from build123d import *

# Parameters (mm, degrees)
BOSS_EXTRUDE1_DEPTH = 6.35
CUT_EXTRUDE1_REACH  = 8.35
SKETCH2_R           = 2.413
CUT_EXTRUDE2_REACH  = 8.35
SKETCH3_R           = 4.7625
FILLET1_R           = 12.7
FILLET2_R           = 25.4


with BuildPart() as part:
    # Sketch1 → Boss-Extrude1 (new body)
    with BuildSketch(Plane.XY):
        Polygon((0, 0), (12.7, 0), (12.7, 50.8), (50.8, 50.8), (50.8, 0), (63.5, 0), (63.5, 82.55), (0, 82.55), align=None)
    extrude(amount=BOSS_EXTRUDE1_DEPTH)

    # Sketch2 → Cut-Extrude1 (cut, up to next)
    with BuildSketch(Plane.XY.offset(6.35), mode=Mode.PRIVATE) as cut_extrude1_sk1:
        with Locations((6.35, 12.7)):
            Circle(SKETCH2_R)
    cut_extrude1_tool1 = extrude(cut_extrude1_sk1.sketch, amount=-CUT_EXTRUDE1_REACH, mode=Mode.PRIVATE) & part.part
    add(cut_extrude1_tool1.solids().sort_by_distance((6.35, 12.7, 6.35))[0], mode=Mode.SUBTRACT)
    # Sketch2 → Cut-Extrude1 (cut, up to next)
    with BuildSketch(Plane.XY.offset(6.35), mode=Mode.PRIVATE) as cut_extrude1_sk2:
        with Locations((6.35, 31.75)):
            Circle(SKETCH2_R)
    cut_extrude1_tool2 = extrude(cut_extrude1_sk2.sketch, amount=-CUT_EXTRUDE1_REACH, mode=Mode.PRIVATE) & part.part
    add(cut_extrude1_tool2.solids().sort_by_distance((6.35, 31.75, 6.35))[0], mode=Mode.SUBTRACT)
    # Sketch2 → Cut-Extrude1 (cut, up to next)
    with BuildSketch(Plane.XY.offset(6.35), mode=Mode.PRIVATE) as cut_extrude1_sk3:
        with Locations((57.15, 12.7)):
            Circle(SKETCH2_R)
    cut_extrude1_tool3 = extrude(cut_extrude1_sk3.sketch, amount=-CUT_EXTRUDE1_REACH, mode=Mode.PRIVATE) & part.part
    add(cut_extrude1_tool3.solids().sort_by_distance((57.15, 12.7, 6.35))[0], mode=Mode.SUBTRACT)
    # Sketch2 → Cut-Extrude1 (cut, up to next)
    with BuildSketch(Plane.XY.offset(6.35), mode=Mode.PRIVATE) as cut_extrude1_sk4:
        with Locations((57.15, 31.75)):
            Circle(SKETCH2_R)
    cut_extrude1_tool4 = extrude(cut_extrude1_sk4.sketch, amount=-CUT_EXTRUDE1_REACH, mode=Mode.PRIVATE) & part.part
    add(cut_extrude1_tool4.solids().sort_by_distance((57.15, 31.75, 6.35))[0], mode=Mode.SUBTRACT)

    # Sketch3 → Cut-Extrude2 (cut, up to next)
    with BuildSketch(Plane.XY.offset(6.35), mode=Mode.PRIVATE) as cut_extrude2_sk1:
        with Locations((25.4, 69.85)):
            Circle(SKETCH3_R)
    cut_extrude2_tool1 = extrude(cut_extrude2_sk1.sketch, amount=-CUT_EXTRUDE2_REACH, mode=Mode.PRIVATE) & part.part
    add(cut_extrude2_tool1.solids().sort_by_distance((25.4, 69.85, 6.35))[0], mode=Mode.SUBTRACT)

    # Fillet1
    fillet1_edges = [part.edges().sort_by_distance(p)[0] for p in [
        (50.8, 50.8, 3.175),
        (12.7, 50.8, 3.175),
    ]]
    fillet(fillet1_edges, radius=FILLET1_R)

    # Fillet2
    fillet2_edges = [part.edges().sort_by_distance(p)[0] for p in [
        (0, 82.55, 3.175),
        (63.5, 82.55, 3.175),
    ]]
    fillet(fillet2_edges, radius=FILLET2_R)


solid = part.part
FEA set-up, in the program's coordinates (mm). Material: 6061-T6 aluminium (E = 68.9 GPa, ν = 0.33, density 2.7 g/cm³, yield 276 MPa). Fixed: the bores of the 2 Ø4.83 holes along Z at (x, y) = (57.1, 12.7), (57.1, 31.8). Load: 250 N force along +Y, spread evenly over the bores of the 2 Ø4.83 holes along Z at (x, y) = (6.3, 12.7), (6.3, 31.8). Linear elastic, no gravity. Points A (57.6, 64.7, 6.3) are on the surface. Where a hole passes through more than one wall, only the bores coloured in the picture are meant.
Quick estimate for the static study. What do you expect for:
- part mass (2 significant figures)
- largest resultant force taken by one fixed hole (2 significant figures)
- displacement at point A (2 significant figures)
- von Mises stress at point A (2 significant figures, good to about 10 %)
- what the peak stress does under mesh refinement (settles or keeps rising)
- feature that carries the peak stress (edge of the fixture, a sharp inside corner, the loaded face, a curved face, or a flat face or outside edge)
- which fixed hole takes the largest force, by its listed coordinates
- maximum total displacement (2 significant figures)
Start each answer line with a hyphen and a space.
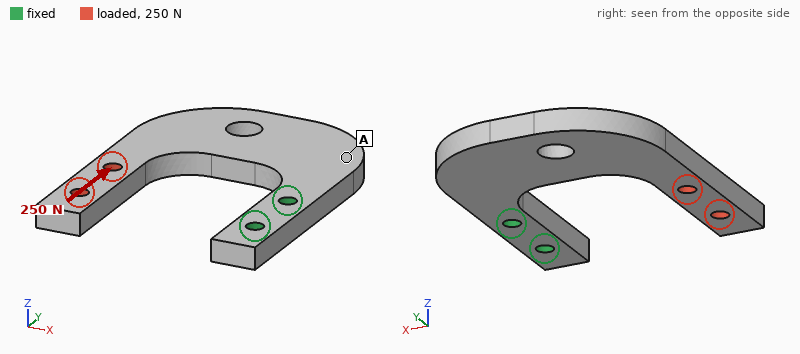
- 51 g
- 350 N
- 0.088 mm
- 9.4 MPa
- keeps rising
- edge of the fixture
- (57.1, 31.8)
- 0.27 mm
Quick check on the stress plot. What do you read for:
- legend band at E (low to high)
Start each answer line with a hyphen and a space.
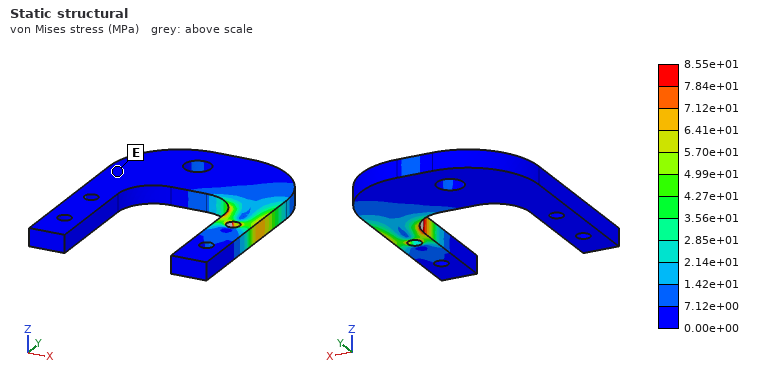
- 0.00e+00 to 7.12e+00 MPa
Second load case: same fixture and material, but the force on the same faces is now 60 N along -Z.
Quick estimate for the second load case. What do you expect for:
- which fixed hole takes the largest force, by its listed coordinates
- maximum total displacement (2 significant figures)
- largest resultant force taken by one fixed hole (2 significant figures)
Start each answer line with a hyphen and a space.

- (57.1, 31.8)
- 0.48 mm
- 57 N
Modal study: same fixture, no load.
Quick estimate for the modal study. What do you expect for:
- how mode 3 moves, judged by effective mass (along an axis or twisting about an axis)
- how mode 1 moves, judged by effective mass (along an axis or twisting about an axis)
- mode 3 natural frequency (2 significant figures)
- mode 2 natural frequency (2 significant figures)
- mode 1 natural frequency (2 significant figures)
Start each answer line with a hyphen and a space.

- along Y
- along Z
- 1000 Hz
- 860 Hz
- 580 Hz
